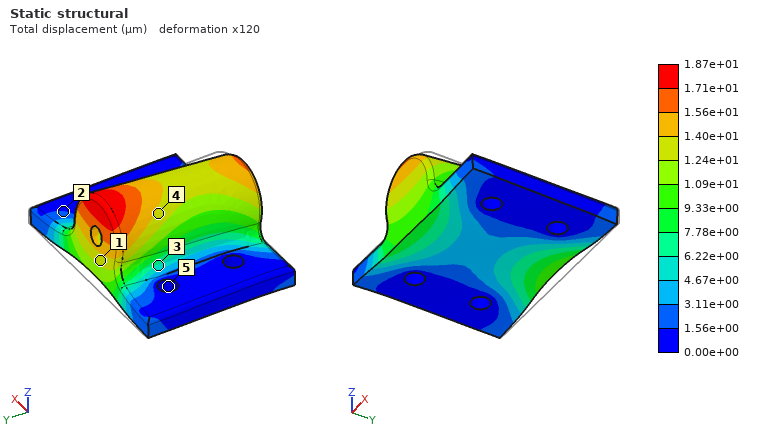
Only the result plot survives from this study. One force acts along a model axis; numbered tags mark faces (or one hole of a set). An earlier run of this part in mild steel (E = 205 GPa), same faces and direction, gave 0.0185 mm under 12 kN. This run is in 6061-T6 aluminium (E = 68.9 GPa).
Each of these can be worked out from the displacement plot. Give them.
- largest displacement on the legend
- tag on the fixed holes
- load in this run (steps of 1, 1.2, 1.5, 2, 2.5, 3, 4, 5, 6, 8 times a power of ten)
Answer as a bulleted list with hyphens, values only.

- 1.87e+01 µm
- 5
- 4 kN
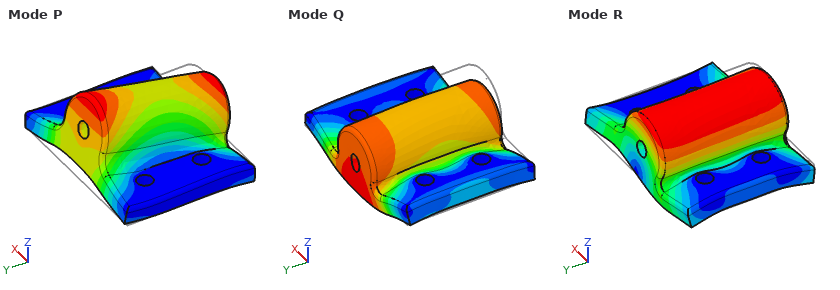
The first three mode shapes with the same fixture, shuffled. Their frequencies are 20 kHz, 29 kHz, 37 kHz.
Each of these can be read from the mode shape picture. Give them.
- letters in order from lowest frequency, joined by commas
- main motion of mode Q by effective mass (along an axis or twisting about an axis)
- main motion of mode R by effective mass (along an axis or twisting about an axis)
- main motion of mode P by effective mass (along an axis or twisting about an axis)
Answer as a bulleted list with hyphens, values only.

- P, Q, R
- along Z
- along X
- along Y
